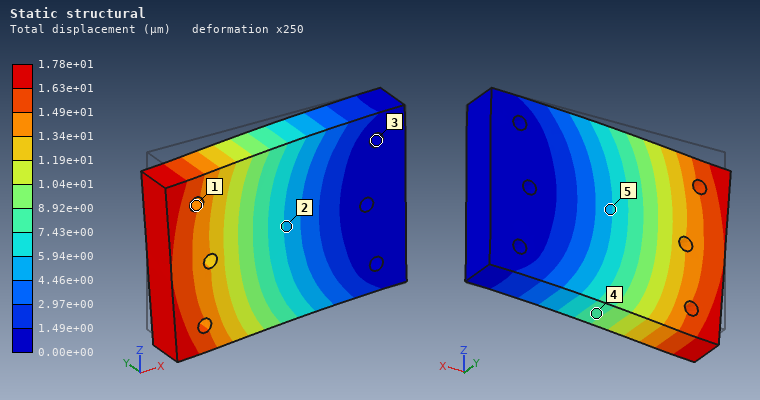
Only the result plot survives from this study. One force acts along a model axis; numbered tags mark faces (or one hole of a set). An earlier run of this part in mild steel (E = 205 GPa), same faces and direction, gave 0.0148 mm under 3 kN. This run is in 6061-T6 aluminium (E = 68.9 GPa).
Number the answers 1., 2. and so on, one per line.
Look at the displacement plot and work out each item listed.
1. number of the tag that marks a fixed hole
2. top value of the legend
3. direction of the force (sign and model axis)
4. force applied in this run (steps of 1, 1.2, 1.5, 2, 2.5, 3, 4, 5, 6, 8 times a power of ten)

1. 3
2. 1.78e+01 µm
3. -Z
4. 1.2 kN
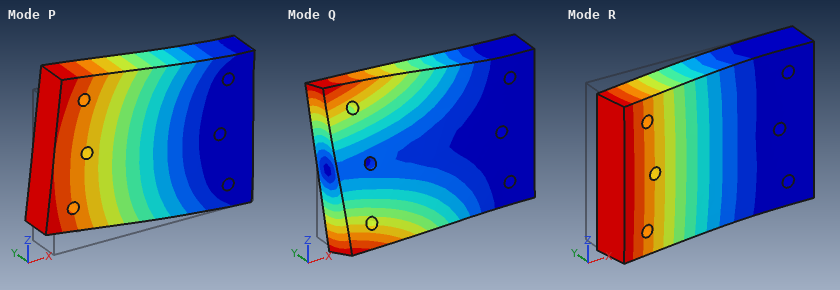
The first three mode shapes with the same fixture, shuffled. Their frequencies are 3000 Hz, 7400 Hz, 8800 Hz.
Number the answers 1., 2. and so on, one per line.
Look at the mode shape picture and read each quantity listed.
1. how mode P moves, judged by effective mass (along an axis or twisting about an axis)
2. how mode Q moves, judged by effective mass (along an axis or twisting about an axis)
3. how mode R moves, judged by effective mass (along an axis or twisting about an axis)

1. along Z
2. twisting about X
3. along Y
